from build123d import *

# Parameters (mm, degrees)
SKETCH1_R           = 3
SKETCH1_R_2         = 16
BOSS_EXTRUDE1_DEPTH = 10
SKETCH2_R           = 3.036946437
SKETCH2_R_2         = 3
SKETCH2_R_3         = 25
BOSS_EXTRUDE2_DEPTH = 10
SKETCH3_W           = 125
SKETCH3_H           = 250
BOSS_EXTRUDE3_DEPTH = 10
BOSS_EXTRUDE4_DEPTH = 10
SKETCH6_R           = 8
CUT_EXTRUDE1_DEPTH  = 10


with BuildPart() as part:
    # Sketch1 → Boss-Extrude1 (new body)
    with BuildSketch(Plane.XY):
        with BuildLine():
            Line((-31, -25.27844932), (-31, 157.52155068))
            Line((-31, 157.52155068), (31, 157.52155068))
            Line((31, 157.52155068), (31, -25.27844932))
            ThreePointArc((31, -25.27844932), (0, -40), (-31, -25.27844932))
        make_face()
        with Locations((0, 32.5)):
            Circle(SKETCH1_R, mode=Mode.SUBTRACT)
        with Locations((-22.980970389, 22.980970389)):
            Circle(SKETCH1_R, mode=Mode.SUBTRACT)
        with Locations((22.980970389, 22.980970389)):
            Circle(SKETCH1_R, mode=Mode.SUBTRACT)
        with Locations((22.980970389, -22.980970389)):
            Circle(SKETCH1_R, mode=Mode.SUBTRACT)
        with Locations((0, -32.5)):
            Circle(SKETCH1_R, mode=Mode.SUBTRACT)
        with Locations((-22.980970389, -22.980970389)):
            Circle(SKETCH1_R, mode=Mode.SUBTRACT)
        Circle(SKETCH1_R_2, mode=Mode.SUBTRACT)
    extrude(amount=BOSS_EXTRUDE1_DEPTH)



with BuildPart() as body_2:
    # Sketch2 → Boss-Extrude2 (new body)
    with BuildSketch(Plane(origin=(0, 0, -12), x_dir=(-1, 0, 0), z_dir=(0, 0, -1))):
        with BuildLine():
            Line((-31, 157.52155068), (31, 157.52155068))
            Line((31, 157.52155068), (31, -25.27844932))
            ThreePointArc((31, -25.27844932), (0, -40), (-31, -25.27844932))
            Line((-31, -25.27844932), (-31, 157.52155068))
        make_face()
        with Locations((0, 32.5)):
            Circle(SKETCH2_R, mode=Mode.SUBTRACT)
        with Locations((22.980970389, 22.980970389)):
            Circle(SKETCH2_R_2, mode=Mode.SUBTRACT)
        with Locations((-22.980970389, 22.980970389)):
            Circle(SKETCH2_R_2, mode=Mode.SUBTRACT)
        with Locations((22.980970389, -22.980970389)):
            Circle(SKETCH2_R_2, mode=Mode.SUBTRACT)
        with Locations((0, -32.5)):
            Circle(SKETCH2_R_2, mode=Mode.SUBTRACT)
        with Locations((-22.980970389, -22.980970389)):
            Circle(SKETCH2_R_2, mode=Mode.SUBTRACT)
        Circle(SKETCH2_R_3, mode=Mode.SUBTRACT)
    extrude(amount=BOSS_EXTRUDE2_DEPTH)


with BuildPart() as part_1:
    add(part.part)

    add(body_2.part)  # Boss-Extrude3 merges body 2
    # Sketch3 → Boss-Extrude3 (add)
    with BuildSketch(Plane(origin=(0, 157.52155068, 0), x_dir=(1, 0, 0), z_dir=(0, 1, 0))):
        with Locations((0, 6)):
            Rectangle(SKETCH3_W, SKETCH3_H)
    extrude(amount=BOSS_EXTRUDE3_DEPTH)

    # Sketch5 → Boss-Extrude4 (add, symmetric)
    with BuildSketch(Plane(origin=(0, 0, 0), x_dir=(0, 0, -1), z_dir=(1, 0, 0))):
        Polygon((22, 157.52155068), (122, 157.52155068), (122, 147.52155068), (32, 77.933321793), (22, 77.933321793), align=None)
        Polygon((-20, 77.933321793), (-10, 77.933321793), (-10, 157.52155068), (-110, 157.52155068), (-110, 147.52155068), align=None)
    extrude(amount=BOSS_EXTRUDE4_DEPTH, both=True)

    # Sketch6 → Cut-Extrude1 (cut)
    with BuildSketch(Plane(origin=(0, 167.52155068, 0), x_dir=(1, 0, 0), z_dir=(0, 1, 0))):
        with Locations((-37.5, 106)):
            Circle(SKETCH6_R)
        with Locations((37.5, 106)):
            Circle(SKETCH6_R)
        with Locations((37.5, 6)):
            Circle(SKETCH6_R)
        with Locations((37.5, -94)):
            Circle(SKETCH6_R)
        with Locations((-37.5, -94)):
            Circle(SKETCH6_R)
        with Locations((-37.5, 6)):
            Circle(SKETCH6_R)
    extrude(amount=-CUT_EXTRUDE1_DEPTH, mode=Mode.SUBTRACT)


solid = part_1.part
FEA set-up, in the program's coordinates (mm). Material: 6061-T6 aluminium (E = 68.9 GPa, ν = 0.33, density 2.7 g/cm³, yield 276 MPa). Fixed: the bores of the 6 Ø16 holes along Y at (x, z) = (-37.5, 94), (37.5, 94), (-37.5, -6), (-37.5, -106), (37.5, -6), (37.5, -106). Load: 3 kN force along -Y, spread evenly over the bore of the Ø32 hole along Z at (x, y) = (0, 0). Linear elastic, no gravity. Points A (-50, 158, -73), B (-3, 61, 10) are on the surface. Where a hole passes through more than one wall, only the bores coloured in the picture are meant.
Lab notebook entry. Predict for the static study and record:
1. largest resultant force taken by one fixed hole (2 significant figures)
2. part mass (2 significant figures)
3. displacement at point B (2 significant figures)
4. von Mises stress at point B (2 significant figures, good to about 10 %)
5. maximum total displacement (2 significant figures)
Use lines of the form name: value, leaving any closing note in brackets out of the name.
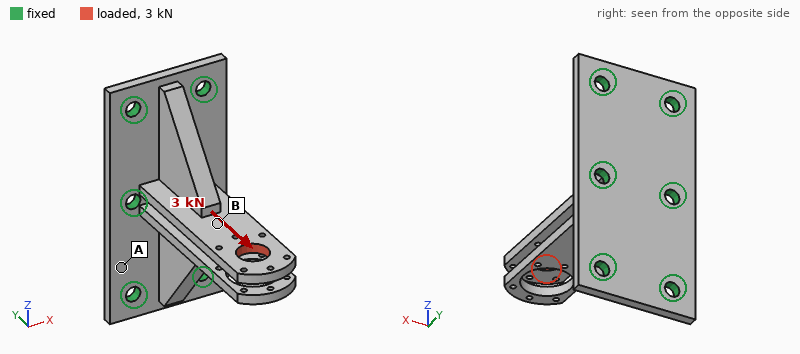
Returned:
largest resultant force taken by one fixed hole: 1.5 kN
part mass: 1.9 kg
displacement at point B: 13 µm
von Mises stress at point B: 4.7 MPa
maximum total displacement: 33 µm
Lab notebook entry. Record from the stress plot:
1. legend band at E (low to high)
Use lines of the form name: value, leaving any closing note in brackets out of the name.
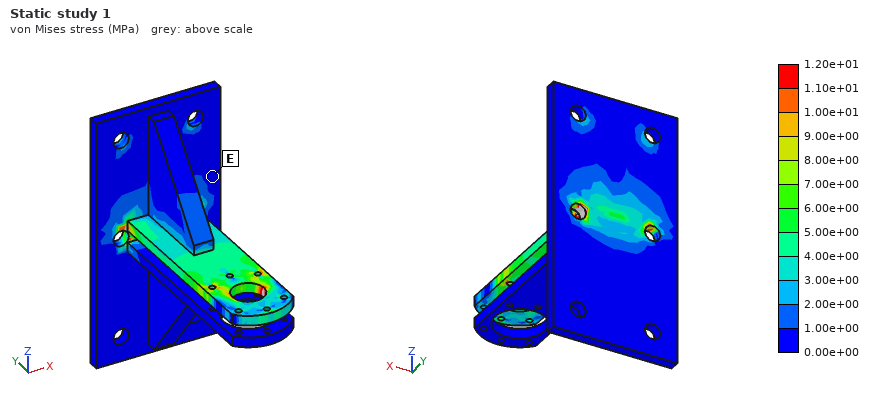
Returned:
legend band at E: 0.00e+00 to 1.00e+00 MPa
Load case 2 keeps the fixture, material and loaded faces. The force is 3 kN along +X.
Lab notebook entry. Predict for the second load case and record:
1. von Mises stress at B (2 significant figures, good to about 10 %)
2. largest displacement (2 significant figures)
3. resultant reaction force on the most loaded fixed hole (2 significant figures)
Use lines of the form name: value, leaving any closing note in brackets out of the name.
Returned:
von Mises stress at B: 13 MPa
largest displacement: 0.51 mm
resultant reaction force on the most loaded fixed hole: 7.2 kN
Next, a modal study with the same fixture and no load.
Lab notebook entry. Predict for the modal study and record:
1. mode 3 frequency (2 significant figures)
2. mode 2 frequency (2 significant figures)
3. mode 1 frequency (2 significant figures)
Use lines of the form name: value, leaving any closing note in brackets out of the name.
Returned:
mode 3 frequency: 1200 Hz
mode 2 frequency: 640 Hz
mode 1 frequency: 580 Hz
